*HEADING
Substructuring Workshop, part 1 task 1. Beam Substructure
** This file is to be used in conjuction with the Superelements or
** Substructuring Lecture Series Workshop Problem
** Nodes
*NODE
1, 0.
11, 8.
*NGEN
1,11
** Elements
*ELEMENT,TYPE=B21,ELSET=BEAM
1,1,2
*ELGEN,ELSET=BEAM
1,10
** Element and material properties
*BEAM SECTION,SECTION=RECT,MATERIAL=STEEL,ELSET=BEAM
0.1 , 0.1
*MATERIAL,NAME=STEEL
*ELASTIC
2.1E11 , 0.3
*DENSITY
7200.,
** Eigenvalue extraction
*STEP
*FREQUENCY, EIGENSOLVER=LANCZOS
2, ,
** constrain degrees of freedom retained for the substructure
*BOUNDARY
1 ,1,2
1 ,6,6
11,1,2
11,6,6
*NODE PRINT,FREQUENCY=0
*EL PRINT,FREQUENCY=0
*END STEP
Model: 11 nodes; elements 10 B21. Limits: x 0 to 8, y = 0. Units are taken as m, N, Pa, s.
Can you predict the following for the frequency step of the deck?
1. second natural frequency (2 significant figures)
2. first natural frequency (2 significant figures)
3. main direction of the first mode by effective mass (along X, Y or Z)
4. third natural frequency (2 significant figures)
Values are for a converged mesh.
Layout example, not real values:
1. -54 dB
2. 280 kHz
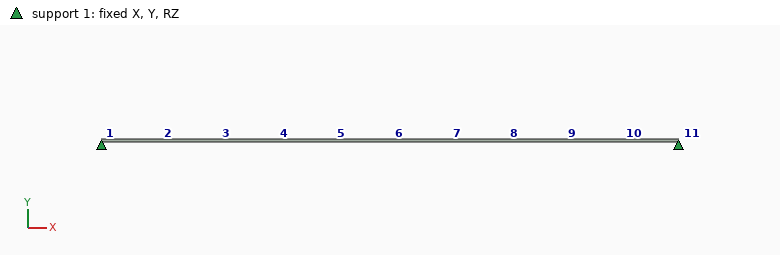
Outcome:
1. 24 Hz
2. 8.7 Hz
3. along Y
4. 47 Hz
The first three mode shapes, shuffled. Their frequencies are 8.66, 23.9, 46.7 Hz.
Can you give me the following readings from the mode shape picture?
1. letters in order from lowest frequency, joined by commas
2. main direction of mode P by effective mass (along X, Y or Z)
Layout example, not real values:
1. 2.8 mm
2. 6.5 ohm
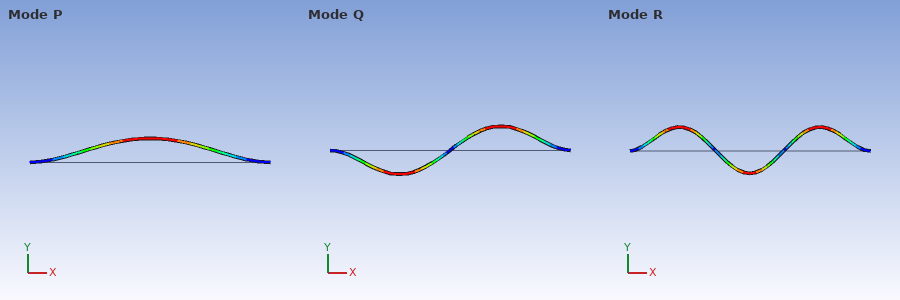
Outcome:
1. P, Q, R
2. along Y
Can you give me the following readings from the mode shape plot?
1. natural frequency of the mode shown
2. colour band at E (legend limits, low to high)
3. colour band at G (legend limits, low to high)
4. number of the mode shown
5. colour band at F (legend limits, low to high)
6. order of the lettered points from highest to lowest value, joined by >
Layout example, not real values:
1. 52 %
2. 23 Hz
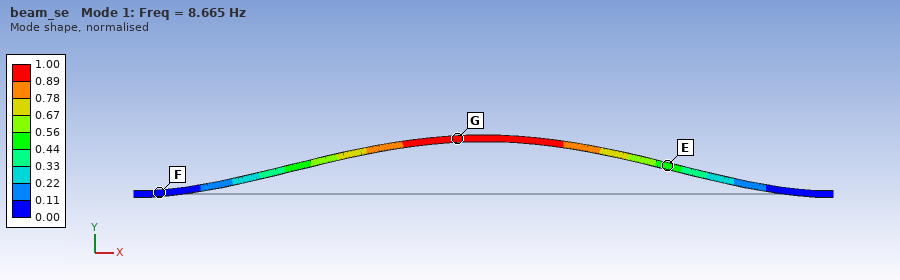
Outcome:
1. 8.665 Hz
2. 0.44 to 0.56
3. 0.89 to 1.00
4. 1
5. 0.00 to 0.11
6. G > E > F
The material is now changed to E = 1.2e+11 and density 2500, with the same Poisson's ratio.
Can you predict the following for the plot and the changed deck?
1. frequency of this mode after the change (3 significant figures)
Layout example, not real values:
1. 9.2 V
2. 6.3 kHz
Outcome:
1. 11.1 Hz
